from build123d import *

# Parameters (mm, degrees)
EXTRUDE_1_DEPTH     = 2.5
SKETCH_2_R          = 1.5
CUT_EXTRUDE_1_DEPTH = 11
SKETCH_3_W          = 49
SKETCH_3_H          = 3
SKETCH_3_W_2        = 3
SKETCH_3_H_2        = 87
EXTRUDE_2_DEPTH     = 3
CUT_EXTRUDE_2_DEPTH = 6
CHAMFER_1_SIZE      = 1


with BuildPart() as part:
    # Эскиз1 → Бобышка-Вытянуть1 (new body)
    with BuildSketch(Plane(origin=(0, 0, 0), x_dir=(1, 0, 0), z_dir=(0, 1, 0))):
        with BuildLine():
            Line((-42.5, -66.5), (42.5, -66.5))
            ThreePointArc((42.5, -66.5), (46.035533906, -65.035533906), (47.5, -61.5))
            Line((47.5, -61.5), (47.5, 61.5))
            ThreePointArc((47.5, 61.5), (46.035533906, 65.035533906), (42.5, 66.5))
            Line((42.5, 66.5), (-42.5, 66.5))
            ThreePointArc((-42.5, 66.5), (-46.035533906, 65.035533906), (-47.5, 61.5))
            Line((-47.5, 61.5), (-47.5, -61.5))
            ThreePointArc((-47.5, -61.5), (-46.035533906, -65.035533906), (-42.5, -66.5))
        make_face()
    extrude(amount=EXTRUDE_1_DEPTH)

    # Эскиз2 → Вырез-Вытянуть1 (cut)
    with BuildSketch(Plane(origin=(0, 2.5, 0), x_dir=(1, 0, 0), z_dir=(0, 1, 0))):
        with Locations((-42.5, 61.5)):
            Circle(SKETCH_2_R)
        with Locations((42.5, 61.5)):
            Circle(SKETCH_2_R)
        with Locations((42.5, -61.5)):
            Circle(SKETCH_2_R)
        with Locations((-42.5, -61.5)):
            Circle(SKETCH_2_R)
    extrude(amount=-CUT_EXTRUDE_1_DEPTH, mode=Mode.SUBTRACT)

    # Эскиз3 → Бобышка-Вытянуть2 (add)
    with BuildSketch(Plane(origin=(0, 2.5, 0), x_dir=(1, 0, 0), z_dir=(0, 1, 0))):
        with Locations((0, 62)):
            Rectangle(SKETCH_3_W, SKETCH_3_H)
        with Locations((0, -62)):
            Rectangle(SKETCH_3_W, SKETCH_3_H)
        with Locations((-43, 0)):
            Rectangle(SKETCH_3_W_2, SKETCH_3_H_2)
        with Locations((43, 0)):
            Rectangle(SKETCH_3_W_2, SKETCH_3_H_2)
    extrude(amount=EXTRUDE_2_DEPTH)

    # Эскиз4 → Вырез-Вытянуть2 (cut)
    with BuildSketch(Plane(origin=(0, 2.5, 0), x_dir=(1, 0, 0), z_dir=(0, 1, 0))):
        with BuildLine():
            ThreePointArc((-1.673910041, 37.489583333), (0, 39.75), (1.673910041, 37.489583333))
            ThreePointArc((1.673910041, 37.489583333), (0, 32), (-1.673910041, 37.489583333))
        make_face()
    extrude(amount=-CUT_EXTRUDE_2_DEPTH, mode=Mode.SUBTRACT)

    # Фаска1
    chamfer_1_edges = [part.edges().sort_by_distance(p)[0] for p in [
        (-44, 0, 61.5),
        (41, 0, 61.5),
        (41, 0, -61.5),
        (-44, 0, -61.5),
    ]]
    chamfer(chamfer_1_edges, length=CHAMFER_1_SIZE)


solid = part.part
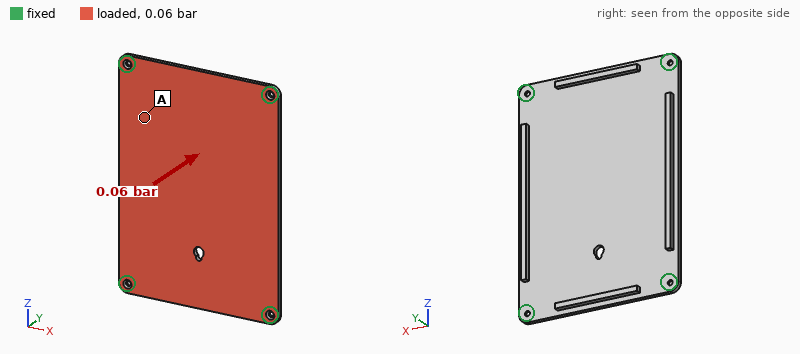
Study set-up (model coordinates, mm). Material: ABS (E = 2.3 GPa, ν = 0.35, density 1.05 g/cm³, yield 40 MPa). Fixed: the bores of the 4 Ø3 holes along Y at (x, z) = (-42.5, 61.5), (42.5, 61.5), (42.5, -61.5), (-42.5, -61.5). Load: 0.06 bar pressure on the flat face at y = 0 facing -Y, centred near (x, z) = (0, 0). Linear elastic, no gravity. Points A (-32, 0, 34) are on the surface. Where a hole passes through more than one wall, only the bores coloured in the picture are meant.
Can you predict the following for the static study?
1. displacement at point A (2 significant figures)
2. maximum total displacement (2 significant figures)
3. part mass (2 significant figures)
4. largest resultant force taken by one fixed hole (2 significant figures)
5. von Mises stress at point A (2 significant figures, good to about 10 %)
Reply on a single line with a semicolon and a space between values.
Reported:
0.92 mm; 1.7 mm; 35 g; 20 N; 1.7 MPa
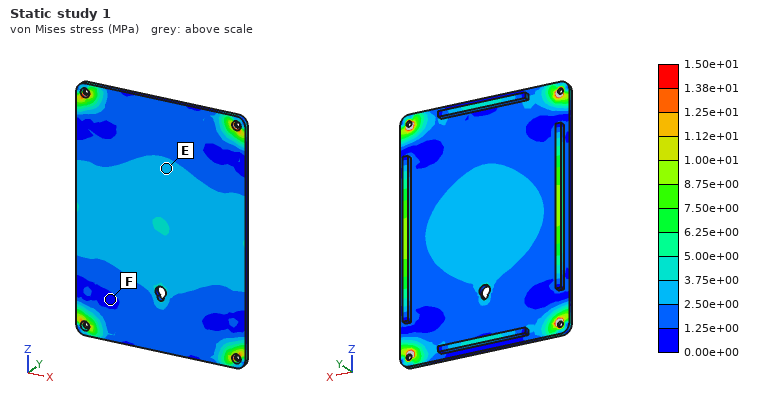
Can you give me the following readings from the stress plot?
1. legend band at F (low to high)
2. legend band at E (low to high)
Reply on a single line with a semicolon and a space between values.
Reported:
0.00e+00 to 1.25e+00 MPa; 2.50e+00 to 3.75e+00 MPa
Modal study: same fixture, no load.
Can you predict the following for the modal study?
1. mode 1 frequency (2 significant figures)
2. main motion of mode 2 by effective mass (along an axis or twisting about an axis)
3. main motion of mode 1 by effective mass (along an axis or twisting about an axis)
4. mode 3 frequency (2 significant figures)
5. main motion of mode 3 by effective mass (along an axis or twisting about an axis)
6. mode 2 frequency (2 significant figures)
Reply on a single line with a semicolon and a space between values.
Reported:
210 Hz; twisting about Z; along Y; 500 Hz; twisting about X; 350 Hz
